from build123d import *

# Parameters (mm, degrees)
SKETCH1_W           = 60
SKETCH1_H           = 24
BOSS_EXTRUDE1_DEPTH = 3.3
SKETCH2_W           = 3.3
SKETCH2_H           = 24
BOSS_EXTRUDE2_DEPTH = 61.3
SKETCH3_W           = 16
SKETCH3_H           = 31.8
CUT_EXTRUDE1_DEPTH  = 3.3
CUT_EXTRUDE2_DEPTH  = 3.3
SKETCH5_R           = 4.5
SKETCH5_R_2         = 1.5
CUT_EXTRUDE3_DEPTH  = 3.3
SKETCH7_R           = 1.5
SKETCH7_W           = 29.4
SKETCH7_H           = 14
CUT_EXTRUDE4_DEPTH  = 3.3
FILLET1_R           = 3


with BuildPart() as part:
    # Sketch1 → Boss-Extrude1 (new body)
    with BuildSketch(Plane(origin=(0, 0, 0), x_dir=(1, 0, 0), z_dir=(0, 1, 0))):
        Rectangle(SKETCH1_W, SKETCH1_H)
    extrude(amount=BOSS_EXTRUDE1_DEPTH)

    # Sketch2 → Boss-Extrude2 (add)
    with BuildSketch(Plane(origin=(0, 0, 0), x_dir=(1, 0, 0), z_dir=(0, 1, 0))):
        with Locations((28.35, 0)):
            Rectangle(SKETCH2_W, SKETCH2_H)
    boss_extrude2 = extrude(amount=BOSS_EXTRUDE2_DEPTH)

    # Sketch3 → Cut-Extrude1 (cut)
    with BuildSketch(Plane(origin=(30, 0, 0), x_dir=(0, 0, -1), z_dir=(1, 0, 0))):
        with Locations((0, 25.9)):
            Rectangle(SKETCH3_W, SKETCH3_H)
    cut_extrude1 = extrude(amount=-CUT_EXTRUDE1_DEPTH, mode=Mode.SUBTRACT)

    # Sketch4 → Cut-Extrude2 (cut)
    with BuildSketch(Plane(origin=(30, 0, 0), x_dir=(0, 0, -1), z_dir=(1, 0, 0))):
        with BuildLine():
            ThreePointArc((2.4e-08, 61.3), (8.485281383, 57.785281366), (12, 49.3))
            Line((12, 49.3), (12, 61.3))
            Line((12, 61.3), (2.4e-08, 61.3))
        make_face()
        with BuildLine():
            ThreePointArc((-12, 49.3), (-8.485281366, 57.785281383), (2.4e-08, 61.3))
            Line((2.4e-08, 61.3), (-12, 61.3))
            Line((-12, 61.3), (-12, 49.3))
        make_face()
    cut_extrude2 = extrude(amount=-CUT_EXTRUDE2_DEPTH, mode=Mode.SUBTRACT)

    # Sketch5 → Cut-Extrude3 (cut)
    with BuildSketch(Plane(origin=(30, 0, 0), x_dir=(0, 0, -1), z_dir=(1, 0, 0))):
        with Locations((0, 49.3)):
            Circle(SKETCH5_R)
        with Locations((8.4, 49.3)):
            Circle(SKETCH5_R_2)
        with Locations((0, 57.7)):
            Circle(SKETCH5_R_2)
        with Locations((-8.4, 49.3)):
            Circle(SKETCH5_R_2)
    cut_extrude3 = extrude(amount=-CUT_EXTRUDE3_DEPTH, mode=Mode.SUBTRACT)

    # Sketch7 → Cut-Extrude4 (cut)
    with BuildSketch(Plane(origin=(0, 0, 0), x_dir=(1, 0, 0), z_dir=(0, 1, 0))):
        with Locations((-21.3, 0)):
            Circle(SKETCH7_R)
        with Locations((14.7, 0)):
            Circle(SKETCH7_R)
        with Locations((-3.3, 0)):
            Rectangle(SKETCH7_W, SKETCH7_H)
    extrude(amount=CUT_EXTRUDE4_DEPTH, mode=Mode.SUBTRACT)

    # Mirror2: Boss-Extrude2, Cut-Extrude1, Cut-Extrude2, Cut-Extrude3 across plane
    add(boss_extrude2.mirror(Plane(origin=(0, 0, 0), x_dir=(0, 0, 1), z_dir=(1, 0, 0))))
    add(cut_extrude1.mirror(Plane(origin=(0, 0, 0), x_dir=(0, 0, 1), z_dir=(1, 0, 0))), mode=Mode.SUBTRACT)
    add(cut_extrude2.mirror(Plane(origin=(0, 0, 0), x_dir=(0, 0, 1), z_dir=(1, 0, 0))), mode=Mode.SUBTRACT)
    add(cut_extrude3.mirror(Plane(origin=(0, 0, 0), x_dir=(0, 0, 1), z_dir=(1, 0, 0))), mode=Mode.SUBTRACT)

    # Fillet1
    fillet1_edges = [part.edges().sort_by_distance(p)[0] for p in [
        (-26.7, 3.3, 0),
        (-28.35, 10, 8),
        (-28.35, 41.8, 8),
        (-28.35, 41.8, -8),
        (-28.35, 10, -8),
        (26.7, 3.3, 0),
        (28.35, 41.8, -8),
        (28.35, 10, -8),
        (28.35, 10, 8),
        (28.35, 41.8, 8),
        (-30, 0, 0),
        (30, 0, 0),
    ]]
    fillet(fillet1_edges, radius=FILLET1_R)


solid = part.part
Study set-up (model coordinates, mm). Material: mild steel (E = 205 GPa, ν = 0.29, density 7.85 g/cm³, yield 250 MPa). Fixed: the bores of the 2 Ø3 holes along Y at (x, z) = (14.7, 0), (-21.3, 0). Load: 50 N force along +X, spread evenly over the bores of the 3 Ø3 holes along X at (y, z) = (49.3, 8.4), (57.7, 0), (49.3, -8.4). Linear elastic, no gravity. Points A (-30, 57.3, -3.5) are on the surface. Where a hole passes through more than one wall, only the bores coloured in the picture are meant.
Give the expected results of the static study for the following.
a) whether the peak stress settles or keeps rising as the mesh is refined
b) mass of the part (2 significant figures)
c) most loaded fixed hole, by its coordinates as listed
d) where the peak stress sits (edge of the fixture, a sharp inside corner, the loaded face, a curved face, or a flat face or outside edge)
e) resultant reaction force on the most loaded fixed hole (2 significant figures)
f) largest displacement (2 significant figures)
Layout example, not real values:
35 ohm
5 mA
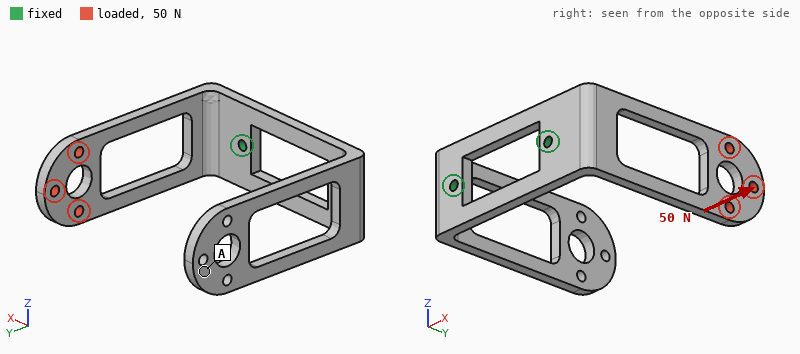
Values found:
keeps rising
65 g
(14.7, 0)
edge of the fixture
53 N
0.55 mm
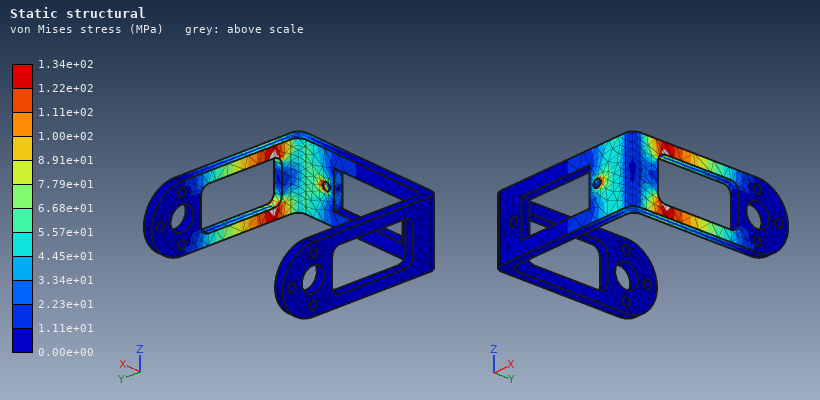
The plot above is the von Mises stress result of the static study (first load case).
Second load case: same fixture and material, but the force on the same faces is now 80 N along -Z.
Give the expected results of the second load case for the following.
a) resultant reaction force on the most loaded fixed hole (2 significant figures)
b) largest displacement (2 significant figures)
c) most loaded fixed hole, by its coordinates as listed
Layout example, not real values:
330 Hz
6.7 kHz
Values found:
88 N
0.19 mm
(14.7, 0)
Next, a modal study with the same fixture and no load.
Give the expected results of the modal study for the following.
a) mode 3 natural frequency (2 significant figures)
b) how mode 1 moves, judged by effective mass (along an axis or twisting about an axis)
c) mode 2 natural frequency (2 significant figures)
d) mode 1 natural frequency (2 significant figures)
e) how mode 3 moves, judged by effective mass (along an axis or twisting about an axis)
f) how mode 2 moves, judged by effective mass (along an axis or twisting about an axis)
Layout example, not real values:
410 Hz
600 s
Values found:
1100 Hz
along X
620 Hz
570 Hz
along Z
along X
